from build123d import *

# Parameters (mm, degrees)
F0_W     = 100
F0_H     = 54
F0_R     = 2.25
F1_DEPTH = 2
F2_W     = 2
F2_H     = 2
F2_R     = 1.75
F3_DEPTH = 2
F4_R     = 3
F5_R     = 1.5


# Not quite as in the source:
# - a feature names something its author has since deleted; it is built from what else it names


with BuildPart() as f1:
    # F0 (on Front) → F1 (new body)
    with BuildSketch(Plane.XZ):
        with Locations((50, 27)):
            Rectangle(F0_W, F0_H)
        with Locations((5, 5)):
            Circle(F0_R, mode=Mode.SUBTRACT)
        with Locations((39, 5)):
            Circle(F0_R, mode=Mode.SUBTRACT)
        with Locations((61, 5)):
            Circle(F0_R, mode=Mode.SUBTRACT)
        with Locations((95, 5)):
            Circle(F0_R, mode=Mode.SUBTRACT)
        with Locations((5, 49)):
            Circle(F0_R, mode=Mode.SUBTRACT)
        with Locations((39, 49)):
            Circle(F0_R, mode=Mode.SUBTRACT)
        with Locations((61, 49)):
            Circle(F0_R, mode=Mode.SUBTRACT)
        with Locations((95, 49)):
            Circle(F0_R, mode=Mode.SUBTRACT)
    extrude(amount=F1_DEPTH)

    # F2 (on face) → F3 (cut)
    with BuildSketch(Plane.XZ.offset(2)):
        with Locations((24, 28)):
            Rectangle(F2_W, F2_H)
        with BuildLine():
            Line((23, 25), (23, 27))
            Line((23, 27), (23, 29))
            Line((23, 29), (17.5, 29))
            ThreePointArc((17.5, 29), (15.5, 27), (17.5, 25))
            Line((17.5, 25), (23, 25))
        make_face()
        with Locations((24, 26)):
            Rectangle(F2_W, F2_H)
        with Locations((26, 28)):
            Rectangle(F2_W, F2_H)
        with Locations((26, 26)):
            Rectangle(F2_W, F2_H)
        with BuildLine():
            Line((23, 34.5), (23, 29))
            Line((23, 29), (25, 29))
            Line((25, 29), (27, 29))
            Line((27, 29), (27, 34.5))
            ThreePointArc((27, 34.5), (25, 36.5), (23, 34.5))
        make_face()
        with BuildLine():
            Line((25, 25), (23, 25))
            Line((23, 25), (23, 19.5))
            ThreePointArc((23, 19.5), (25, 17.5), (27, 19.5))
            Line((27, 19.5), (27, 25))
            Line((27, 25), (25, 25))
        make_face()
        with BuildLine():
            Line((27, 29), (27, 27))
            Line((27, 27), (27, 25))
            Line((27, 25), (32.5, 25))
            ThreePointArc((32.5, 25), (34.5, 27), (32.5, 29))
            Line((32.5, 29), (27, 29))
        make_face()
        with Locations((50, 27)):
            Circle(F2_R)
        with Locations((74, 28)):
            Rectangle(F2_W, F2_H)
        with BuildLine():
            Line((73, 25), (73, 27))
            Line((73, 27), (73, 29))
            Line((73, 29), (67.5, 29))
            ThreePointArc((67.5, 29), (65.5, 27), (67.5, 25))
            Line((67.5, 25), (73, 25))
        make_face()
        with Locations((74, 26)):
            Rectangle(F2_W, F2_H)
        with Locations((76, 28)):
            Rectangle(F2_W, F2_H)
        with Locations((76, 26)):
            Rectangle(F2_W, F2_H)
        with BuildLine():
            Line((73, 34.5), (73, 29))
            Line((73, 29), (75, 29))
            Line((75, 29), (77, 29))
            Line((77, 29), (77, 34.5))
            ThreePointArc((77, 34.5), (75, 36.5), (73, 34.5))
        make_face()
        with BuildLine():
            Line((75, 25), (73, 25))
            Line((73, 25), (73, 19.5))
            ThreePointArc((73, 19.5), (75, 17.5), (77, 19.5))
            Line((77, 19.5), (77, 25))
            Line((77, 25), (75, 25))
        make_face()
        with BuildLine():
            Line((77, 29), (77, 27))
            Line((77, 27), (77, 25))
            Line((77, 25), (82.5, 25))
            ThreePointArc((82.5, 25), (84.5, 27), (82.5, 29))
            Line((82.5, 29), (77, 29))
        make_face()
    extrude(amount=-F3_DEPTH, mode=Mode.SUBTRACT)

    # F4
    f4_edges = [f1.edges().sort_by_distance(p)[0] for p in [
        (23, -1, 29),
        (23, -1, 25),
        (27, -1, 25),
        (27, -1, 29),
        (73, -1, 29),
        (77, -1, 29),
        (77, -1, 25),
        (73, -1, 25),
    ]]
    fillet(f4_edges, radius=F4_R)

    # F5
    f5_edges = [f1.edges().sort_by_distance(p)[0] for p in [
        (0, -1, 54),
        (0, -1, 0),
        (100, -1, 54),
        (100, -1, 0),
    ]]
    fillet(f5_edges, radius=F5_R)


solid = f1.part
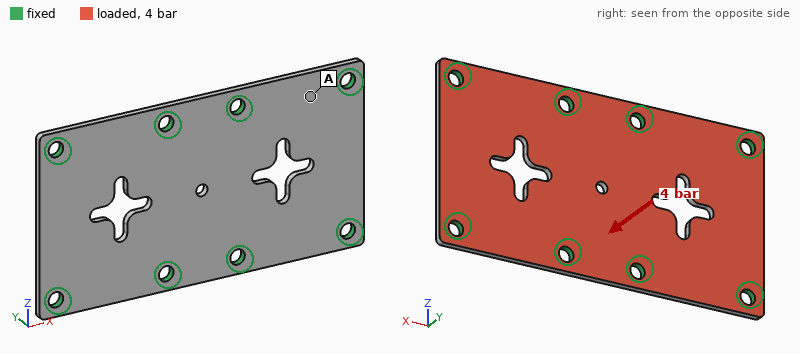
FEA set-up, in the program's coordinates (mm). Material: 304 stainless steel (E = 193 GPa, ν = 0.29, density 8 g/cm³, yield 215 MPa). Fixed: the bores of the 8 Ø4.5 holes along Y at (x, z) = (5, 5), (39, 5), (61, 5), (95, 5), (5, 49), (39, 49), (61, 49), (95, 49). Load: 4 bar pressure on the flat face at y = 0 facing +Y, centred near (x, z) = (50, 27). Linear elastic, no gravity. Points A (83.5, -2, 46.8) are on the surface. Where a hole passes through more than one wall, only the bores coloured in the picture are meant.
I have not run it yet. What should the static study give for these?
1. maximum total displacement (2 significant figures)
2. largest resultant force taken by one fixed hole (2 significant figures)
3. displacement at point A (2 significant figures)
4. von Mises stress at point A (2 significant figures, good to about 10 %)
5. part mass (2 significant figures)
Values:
49 µm
280 N
11 µm
32 MPa
80 g
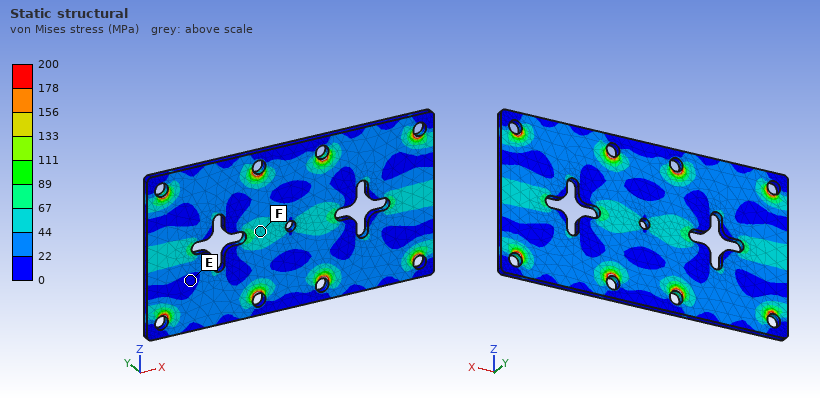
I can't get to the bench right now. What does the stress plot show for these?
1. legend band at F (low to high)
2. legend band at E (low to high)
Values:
44 to 67 MPa
0 to 22 MPa
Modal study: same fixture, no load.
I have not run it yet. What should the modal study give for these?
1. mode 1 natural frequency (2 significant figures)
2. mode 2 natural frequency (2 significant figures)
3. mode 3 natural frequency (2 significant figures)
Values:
4800 Hz
4900 Hz
6200 Hz
